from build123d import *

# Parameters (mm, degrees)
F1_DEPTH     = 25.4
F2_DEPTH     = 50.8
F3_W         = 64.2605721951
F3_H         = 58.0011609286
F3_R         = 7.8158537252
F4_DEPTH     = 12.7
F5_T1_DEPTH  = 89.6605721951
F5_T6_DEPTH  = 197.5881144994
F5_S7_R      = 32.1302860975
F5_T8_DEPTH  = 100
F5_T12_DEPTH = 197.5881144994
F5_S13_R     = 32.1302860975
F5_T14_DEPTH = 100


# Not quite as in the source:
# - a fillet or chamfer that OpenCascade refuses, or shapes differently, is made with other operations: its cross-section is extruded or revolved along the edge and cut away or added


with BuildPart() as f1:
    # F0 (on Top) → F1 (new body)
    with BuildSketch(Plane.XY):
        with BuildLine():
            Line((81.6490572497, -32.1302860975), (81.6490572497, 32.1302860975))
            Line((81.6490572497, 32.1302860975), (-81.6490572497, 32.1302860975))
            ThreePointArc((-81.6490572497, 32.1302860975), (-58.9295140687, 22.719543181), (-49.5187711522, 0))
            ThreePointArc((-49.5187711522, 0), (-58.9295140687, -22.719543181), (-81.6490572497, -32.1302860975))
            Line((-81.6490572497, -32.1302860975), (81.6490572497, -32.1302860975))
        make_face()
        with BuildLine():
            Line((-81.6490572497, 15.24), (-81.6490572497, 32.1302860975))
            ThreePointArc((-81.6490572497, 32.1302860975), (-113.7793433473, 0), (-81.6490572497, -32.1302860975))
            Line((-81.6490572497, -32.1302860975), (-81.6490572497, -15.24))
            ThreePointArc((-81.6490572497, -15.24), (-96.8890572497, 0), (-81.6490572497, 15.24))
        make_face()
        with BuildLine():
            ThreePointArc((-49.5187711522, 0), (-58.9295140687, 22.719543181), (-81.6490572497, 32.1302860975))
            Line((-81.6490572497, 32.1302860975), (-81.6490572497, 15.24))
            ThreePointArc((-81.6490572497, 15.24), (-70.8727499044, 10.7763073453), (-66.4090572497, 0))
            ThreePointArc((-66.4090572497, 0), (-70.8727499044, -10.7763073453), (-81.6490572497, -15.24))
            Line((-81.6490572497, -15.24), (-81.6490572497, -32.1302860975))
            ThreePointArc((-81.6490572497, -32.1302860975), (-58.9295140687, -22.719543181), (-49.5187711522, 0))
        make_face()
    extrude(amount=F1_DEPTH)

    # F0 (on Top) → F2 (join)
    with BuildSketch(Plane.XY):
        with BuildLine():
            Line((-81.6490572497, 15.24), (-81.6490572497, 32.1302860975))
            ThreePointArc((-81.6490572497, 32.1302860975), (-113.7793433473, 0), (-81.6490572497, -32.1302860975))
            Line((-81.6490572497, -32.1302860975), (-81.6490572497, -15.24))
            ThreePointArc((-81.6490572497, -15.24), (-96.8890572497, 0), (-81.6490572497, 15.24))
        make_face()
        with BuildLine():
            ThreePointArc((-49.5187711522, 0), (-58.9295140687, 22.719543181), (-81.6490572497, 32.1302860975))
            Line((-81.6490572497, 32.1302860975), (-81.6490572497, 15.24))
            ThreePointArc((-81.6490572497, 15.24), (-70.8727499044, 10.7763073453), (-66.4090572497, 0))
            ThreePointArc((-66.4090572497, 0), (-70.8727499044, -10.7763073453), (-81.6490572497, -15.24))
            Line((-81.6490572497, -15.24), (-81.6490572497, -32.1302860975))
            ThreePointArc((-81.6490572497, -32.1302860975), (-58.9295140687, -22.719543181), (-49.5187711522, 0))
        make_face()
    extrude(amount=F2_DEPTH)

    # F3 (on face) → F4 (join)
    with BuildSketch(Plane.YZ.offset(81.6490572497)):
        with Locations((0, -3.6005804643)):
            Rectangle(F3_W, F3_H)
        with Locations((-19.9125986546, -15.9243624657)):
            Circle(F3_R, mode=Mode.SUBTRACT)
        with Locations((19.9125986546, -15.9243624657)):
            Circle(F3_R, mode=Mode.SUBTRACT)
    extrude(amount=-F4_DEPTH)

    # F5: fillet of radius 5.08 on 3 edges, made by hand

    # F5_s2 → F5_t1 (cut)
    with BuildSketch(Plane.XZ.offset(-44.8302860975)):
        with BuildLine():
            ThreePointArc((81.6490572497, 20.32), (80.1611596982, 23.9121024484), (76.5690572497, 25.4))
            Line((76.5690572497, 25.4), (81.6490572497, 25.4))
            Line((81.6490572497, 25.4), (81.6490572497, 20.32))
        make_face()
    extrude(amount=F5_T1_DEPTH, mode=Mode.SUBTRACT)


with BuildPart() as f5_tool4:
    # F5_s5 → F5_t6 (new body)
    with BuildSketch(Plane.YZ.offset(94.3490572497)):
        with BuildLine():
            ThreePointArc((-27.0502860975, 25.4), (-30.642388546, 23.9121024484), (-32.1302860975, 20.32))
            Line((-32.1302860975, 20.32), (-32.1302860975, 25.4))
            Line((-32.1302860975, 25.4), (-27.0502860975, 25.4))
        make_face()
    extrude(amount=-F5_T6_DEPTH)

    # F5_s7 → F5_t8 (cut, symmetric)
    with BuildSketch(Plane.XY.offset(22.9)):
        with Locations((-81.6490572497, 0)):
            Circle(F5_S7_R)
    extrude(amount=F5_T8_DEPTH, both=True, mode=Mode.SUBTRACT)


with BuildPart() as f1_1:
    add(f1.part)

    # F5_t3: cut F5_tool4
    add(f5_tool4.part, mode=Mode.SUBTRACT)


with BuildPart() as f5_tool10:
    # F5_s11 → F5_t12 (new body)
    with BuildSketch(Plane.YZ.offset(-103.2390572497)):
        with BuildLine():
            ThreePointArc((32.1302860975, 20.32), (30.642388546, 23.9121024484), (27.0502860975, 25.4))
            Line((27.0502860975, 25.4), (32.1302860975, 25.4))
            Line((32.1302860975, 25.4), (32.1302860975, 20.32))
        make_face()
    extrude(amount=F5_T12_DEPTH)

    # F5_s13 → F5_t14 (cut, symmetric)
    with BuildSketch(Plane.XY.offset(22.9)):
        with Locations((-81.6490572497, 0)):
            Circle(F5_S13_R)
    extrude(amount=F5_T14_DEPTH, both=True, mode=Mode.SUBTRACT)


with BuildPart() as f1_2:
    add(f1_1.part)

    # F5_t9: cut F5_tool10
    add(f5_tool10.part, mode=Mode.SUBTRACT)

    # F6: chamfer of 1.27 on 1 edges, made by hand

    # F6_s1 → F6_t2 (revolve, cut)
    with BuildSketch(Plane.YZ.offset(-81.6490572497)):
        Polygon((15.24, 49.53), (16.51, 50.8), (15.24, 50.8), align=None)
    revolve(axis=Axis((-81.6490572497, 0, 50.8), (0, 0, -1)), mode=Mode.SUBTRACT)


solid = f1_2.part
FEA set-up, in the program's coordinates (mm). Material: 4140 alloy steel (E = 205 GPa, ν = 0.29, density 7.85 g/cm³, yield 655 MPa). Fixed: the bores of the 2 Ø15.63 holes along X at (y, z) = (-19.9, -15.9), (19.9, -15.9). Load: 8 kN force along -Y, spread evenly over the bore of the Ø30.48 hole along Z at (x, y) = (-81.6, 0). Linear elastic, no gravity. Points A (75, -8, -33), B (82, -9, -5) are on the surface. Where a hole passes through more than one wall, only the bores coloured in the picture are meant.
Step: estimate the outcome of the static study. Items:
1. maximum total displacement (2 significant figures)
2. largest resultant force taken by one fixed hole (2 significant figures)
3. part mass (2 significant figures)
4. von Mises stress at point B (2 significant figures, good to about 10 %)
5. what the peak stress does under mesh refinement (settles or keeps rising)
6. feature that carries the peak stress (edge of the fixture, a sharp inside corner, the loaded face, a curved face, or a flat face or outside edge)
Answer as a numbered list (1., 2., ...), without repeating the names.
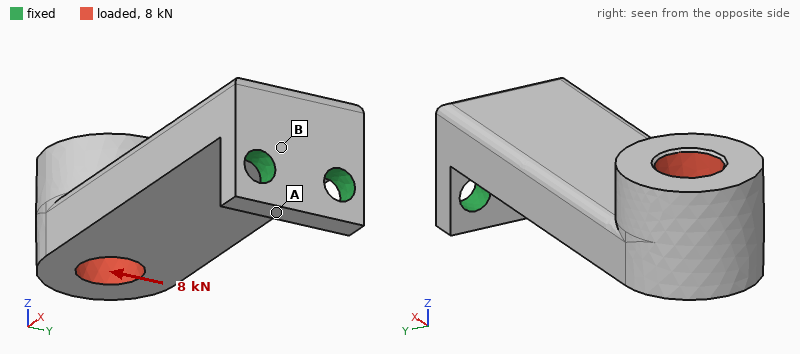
1. 0.41 mm
2. 28 kN
3. 2.9 kg
4. 95 MPa
5. keeps rising
6. edge of the fixture
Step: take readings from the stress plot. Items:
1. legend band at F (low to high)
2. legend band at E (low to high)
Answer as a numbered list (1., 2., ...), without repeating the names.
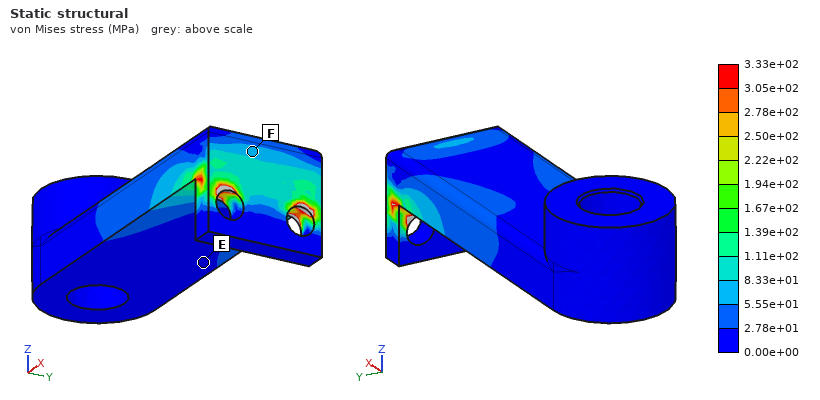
1. 5.55e+01 to 8.33e+01 MPa
2. 0.00e+00 to 2.78e+01 MPa
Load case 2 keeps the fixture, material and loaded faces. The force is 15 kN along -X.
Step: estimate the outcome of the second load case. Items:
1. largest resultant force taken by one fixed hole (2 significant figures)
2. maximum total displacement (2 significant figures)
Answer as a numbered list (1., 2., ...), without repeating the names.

1. 7.5 kN
2. 0.79 mm
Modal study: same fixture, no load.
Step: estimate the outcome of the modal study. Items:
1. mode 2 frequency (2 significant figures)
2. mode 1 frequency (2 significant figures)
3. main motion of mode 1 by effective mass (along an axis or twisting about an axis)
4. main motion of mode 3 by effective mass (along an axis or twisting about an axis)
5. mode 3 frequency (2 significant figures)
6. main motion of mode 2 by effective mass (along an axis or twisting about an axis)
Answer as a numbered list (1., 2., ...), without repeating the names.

1. 660 Hz
2. 270 Hz
3. along Z
4. twisting about X
5. 2100 Hz
6. along Y
